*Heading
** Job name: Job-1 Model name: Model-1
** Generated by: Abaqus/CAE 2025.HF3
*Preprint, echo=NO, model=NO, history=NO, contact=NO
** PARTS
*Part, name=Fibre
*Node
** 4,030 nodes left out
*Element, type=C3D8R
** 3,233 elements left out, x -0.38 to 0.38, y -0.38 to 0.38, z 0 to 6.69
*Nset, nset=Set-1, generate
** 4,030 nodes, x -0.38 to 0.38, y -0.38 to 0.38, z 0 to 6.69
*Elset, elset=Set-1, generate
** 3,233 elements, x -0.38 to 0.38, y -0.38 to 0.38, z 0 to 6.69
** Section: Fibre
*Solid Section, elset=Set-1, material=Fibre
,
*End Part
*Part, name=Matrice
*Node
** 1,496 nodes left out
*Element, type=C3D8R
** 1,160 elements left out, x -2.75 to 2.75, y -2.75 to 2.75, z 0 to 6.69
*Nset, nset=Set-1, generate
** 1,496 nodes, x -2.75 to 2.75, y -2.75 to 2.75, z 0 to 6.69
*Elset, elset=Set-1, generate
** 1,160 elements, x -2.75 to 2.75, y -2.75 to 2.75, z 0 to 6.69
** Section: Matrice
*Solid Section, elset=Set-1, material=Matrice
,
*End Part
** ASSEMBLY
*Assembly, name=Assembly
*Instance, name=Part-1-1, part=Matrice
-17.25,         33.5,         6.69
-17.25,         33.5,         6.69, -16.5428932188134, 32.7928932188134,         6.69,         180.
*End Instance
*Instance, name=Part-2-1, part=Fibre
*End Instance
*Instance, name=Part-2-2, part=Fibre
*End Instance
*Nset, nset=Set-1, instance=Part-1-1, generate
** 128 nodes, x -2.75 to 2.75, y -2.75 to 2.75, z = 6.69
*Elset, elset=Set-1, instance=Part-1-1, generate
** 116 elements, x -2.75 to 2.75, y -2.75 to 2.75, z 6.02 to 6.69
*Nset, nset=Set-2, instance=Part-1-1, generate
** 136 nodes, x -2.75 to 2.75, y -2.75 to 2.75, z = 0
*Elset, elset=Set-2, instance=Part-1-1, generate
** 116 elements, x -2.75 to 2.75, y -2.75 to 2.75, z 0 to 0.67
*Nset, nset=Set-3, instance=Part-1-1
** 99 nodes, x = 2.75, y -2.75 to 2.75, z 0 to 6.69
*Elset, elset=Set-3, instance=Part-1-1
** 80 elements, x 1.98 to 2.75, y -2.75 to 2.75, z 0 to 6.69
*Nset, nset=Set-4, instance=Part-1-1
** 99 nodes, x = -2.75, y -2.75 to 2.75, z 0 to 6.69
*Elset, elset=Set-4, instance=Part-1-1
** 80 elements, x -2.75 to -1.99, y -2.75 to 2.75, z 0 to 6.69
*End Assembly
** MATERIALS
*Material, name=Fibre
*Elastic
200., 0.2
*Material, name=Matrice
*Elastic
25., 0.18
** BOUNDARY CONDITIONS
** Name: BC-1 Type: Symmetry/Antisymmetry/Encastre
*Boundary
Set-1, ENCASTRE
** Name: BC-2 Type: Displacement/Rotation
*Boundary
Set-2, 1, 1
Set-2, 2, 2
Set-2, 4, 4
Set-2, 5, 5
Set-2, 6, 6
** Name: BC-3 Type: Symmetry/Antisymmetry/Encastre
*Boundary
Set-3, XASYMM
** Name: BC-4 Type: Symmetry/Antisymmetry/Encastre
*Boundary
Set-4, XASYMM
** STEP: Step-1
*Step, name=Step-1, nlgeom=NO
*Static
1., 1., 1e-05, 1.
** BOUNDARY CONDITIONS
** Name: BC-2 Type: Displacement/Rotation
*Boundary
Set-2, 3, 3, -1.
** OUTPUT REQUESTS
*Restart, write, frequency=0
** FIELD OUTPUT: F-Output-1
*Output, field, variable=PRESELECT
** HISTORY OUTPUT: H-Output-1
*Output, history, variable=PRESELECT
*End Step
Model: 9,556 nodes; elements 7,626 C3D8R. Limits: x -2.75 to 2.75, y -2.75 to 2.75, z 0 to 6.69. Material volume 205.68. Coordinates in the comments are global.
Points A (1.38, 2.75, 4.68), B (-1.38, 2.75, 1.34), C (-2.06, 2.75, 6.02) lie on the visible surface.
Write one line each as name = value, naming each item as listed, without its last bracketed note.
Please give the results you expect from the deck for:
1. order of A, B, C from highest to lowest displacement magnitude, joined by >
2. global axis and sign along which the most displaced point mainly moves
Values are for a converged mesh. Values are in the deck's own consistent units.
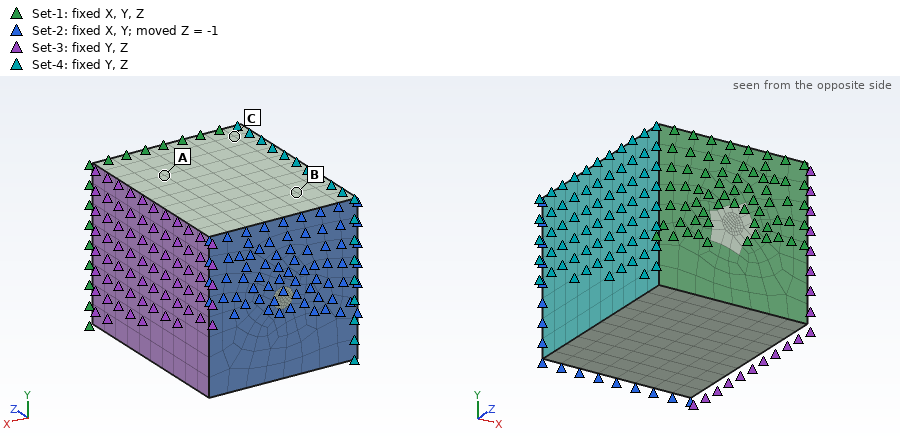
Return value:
order of A, B, C from highest to lowest displacement magnitude, joined by > = B > A > C
global axis and sign along which the most displaced point mainly moves = -Z
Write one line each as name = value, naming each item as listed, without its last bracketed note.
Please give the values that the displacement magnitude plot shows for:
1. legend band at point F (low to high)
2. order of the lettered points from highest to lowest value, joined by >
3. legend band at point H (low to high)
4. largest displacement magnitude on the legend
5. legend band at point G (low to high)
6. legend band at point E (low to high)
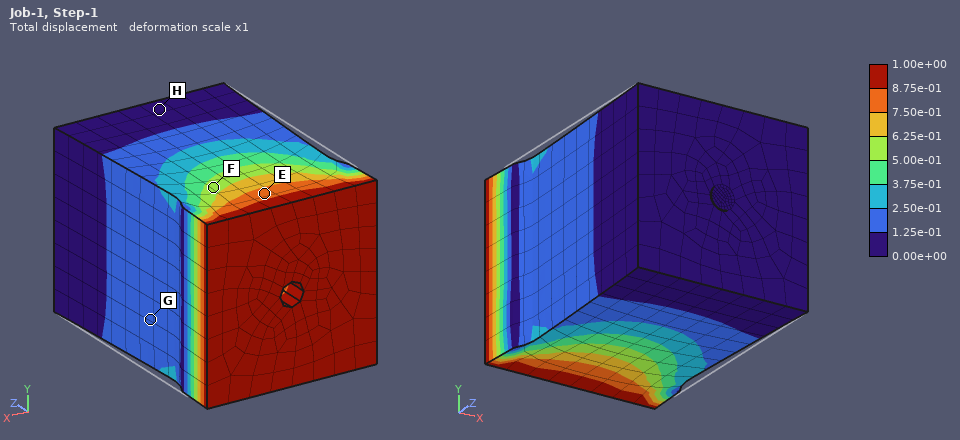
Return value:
legend band at point F = 5.00e-01 to 6.25e-01
order of the lettered points from highest to lowest value, joined by > = E > F > G > H
legend band at point H = 0.00e+00 to 1.25e-01
largest displacement magnitude on the legend = 1.00e+00
legend band at point G = 1.25e-01 to 2.50e-01
legend band at point E = 7.50e-01 to 8.75e-01
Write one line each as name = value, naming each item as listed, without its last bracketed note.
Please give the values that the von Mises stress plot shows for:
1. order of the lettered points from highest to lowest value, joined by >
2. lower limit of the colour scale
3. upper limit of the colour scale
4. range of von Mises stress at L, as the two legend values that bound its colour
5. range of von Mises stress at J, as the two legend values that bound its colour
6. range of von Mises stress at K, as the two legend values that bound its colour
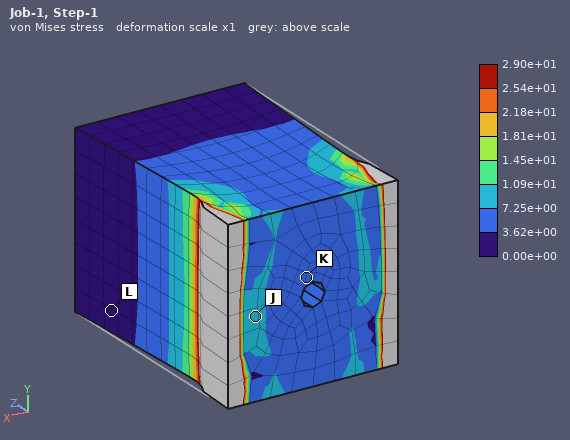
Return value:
order of the lettered points from highest to lowest value, joined by > = J > K > L
lower limit of the colour scale = 0.00e+00
upper limit of the colour scale = 2.90e+01
range of von Mises stress at L, as the two legend values that bound its colour = 0.00e+00 to 3.62e+00
range of von Mises stress at J, as the two legend values that bound its colour = 7.25e+00 to 1.09e+01
range of von Mises stress at K, as the two legend values that bound its colour = 3.62e+00 to 7.25e+00
